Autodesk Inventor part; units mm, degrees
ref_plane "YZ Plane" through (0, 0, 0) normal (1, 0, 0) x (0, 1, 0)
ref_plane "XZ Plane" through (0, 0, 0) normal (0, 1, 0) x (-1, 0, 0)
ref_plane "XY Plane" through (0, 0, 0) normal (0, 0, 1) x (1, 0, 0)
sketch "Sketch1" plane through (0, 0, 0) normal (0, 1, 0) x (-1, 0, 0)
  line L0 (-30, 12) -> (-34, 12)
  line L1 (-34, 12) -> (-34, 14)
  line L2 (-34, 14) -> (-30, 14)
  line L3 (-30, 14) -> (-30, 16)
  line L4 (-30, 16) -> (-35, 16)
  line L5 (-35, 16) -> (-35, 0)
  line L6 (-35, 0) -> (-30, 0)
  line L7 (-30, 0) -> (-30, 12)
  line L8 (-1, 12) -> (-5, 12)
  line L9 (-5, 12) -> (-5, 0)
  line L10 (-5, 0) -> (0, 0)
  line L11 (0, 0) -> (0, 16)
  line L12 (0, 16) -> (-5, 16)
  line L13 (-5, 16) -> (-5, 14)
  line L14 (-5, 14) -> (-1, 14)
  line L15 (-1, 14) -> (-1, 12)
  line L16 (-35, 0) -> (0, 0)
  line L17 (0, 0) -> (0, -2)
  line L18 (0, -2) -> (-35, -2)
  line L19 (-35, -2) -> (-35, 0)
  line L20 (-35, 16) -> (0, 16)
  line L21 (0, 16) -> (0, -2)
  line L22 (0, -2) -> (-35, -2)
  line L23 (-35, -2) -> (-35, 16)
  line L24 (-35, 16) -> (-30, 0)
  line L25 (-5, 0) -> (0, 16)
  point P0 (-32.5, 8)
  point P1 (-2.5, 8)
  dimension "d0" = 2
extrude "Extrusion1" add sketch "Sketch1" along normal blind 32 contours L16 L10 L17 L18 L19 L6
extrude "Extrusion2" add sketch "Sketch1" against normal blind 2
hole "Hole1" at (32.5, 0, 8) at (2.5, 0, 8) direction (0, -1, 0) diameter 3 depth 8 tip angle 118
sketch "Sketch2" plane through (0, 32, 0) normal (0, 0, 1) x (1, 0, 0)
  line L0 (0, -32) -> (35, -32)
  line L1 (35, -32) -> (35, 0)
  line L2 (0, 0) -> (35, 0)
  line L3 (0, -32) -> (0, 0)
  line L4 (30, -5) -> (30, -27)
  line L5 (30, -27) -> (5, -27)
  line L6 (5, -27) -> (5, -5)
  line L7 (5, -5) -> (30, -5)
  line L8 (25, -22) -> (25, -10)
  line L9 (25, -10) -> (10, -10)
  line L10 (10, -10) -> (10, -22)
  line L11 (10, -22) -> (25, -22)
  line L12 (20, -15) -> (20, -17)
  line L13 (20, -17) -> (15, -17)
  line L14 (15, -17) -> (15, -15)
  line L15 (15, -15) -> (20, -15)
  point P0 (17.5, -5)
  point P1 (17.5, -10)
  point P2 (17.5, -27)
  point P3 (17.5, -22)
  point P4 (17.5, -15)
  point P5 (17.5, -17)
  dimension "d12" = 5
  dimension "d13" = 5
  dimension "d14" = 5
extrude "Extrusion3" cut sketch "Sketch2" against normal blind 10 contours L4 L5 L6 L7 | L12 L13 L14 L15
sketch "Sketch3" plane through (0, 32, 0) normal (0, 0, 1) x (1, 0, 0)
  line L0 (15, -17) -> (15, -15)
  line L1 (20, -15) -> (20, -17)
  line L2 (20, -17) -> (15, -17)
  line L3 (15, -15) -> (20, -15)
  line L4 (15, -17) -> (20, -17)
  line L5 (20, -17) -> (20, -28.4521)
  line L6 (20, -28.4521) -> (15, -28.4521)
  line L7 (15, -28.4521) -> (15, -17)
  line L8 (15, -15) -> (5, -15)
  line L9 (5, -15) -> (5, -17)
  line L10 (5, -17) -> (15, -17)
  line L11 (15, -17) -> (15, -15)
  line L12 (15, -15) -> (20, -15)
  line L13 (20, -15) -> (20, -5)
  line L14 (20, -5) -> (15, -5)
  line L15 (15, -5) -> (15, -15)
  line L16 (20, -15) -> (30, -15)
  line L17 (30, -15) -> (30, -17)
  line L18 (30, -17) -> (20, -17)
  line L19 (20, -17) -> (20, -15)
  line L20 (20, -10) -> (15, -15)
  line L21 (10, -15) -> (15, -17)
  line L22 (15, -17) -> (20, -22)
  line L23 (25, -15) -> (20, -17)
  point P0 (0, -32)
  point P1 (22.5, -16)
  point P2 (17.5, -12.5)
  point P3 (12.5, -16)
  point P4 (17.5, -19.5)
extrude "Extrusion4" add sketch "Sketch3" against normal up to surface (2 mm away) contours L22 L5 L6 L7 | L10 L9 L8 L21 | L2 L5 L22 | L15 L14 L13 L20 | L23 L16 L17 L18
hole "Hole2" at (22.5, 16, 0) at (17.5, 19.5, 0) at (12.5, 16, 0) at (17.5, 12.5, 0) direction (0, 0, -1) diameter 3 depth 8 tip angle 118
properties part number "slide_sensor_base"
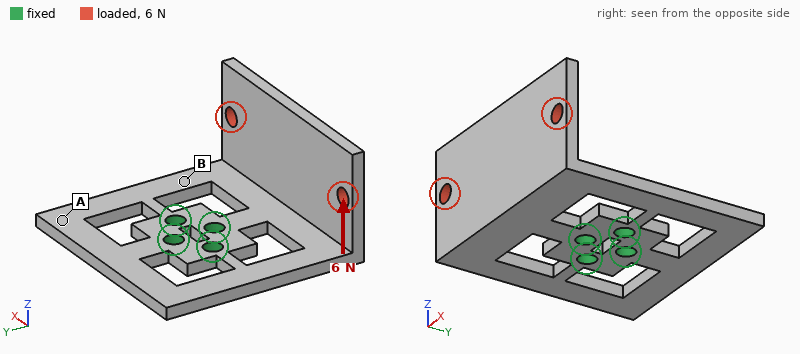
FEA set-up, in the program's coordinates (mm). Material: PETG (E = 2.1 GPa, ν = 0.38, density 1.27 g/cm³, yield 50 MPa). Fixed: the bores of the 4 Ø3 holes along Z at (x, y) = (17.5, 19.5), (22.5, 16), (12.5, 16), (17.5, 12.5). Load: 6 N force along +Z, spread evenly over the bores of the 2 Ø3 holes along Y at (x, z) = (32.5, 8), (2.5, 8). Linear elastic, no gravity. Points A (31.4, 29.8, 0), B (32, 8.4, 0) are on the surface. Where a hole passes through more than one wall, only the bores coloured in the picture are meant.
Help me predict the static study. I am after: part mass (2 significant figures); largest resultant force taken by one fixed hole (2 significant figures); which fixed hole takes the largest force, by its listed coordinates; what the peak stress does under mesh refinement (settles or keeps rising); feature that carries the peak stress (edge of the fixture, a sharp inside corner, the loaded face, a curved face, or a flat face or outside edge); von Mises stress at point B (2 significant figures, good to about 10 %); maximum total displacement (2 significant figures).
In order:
3.5 g
9.5 N
(17.5, 12.5)
keeps rising
edge of the fixture
3.0 MPa
0.60 mm
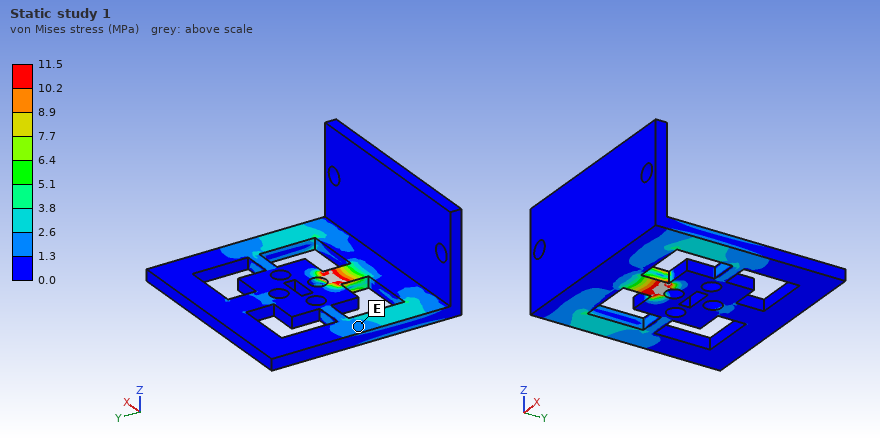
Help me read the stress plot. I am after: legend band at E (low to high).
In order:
1.3 to 2.6 MPa
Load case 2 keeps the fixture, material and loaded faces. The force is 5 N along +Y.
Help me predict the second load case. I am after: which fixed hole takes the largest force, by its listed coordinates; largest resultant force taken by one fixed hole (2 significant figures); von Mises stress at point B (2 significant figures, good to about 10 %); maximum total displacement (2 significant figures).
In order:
(17.5, 12.5)
4.2 N
3.4 MPa
0.55 mm
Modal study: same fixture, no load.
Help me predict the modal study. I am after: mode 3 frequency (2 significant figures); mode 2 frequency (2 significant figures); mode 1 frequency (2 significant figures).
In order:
1100 Hz
480 Hz
390 Hz
